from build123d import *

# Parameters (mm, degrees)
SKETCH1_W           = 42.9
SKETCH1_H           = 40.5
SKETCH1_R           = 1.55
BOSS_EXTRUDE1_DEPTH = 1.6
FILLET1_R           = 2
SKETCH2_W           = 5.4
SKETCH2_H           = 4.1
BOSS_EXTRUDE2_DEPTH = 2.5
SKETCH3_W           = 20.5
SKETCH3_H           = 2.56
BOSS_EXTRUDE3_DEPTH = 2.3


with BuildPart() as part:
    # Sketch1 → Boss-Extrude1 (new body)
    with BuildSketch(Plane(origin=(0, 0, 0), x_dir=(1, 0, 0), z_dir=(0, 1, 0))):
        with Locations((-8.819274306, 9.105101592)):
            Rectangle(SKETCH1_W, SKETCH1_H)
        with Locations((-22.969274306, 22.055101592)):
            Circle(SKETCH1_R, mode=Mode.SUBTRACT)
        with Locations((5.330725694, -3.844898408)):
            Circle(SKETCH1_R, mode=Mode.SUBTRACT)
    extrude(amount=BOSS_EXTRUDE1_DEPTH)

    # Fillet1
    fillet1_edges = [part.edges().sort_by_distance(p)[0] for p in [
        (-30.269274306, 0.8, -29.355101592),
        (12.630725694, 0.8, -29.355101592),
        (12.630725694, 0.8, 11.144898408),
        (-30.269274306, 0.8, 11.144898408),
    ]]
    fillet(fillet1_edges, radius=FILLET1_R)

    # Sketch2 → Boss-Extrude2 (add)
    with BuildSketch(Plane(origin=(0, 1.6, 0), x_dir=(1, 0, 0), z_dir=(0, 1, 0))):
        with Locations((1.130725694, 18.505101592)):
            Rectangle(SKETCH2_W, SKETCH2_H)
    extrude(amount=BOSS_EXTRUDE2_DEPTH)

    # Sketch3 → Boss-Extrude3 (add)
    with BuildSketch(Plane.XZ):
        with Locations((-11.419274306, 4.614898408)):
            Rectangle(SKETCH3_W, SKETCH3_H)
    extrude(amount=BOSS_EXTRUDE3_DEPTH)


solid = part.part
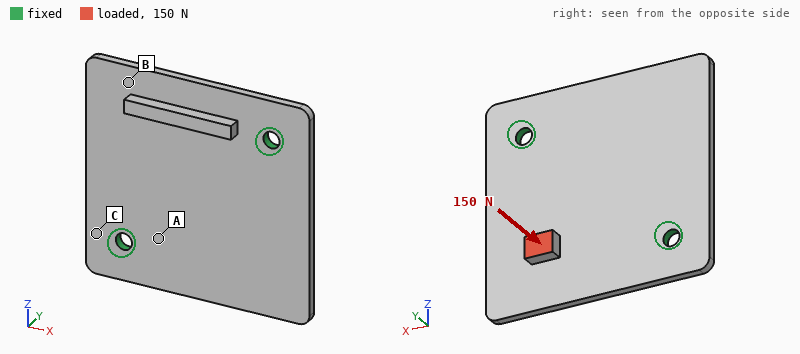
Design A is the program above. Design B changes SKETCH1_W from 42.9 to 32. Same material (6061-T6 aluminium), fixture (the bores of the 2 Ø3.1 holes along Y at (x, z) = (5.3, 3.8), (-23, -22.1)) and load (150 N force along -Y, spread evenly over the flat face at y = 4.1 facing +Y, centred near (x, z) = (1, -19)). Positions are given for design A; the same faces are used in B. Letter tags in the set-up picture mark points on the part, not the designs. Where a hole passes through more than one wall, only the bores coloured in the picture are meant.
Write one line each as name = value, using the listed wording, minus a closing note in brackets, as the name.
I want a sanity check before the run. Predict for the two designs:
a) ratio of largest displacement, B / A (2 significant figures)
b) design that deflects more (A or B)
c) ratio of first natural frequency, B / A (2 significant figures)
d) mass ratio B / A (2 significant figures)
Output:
ratio of largest displacement, B / A = 1.1
design that deflects more = B
ratio of first natural frequency, B / A = 1.1
mass ratio B / A = 0.76
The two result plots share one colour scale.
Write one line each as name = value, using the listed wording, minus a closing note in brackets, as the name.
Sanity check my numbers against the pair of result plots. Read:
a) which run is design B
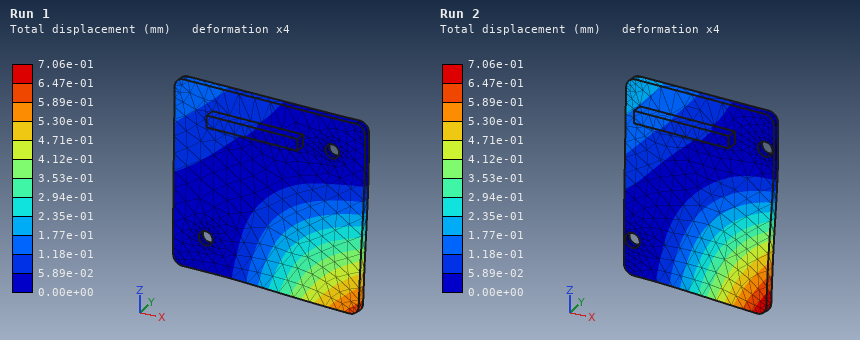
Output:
which run is design B = Run 2
